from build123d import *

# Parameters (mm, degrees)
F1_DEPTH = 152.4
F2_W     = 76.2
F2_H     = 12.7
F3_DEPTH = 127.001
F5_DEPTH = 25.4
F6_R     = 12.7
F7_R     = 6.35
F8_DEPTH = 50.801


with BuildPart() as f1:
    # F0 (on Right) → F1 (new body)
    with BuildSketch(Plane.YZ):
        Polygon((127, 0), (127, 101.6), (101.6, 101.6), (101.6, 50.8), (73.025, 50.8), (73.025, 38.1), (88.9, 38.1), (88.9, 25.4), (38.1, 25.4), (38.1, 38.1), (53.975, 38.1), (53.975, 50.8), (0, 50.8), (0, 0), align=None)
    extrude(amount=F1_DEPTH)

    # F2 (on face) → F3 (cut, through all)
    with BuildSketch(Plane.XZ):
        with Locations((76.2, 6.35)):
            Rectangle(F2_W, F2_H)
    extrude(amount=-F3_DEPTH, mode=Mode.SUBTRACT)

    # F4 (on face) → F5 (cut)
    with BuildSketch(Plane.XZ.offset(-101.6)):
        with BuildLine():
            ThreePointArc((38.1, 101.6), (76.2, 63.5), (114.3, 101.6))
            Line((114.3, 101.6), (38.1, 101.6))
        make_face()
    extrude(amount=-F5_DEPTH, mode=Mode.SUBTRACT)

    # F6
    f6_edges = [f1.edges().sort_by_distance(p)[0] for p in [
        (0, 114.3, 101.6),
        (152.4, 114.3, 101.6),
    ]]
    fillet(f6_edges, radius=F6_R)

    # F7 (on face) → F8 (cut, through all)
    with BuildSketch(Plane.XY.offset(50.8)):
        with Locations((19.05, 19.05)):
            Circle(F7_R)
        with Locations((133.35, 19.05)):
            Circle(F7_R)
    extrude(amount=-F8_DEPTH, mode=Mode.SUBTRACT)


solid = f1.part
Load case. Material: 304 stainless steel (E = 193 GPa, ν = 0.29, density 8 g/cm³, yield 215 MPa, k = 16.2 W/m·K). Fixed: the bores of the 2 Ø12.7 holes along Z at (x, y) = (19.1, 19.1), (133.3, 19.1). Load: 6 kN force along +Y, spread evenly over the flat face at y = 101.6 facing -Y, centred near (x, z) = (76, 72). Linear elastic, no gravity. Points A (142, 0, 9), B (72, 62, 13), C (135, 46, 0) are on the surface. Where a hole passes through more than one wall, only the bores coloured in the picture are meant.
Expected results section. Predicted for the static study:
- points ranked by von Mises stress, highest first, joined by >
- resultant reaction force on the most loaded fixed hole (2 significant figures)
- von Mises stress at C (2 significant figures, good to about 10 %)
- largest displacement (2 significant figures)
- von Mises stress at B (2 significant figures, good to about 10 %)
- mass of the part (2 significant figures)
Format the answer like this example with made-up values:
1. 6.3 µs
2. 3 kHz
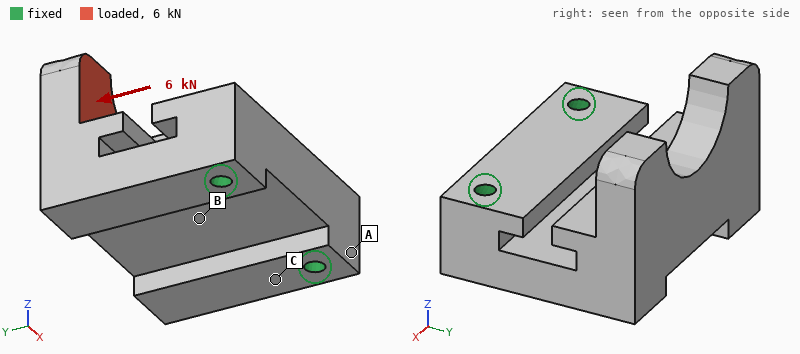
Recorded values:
1. C > B > A
2. 3.4 kN
3. 32 MPa
4. 0.11 mm
5. 14 MPa
6. 6.8 kg
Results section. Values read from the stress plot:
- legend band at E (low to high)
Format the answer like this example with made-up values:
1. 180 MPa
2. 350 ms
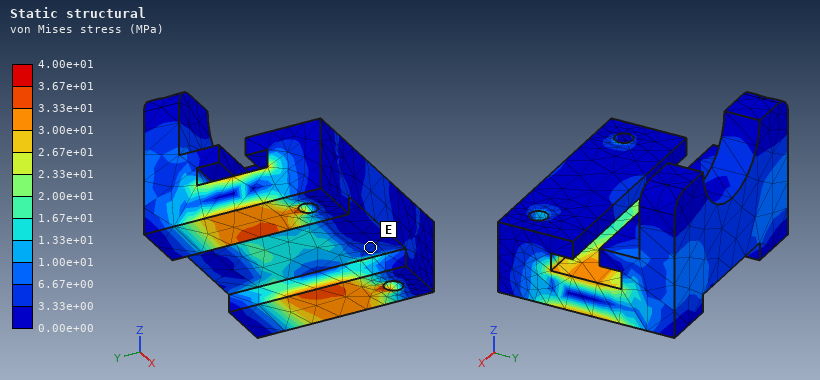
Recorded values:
1. 3.33e+00 to 6.67e+00 MPa
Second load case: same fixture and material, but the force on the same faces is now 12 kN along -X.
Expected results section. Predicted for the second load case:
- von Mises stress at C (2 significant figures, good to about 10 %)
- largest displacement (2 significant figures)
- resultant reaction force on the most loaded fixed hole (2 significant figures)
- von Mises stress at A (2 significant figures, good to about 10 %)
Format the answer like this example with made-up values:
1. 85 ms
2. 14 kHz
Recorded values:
1. 32 MPa
2. 64 µm
3. 11 kN
4. 4.4 MPa
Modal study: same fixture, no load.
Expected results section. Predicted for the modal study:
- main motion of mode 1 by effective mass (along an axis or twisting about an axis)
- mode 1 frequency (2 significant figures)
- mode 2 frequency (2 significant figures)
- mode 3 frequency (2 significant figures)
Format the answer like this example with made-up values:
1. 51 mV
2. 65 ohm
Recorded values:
1. along Z
2. 810 Hz
3. 1600 Hz
4. 2800 Hz
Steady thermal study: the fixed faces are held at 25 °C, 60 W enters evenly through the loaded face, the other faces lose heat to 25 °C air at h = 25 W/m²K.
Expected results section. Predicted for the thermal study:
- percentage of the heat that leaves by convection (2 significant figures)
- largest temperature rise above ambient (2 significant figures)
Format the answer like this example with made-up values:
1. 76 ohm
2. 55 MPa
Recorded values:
1. 78 %
2. 67 K
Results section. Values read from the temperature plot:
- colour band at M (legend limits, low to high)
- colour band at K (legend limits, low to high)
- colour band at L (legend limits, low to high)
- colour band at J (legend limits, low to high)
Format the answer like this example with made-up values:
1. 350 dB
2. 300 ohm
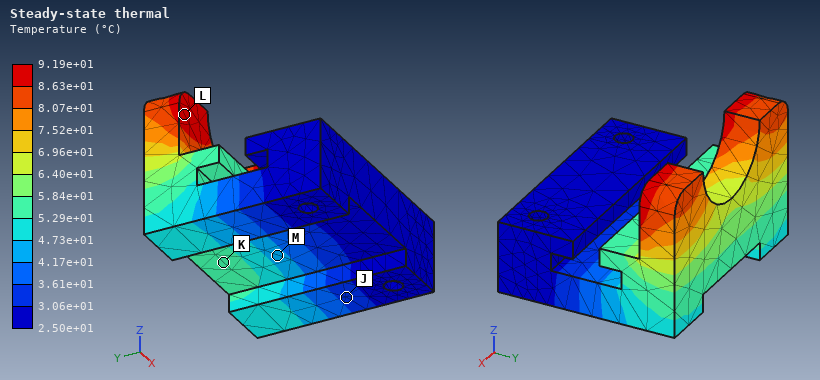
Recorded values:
1. 4.17e+01 to 4.73e+01 °C
2. 5.29e+01 to 5.84e+01 °C
3. 8.63e+01 to 9.19e+01 °C
4. 3.06e+01 to 3.61e+01 °C
